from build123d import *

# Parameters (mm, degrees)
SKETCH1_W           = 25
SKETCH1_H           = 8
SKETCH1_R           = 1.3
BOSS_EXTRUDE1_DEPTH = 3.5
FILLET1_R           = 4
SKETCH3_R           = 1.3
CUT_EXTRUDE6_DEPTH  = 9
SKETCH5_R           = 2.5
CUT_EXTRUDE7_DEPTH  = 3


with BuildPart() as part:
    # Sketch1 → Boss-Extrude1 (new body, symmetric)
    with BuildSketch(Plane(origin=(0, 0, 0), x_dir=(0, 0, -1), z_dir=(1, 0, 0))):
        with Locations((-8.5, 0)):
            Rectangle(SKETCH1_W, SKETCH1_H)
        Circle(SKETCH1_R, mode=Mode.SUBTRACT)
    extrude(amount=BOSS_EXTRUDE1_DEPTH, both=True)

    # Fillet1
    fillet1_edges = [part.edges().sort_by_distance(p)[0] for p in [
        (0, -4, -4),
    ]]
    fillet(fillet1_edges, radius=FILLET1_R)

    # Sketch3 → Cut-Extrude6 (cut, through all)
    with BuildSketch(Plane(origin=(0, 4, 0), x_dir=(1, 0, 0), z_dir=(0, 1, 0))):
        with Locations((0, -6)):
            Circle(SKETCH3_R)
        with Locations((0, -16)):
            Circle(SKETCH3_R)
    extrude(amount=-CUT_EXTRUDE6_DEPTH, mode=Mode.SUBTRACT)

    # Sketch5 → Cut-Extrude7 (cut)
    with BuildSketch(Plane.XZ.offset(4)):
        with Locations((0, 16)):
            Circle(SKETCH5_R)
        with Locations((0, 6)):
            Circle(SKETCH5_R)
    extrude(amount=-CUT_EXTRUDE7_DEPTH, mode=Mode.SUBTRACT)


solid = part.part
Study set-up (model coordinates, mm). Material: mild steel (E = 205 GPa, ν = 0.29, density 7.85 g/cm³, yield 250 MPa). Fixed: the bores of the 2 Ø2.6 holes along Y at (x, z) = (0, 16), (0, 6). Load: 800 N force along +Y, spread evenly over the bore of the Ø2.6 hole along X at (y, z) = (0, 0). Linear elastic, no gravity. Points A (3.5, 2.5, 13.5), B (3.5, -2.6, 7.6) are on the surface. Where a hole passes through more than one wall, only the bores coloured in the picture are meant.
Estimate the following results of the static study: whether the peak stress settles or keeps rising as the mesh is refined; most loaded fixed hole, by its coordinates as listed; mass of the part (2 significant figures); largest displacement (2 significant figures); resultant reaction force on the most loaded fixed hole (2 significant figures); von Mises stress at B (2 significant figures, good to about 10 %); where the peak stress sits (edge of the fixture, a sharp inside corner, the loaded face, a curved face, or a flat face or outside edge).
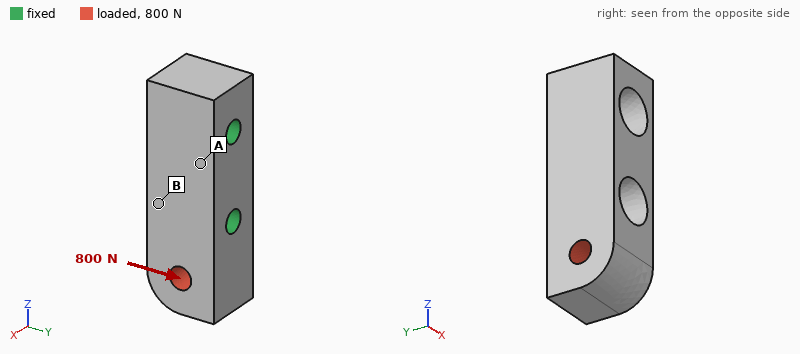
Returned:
keeps rising
(0, 6)
9.2 g
6.2 µm
950 N
45 MPa
edge of the fixture
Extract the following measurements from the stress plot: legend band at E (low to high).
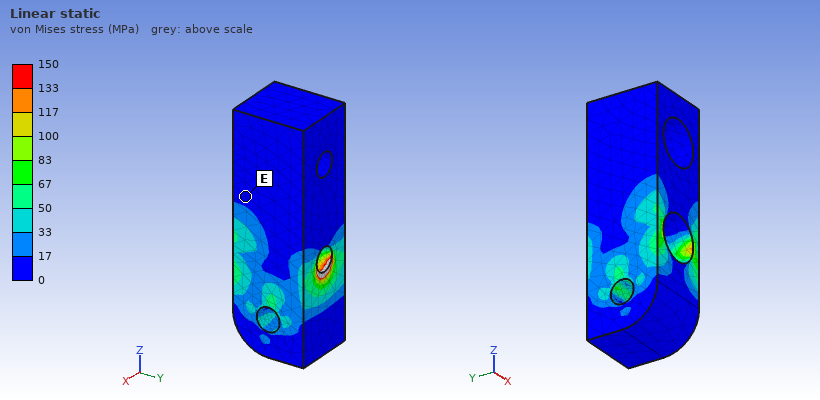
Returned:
0 to 17 MPa
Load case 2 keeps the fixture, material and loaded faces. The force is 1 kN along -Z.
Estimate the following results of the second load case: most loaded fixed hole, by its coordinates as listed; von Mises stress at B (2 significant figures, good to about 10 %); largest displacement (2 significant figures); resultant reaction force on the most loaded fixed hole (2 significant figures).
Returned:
(0, 6)
25 MPa
1.9 µm
860 N
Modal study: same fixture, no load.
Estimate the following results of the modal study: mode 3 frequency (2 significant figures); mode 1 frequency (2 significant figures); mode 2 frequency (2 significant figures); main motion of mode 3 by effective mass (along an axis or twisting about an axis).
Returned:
59 kHz
37 kHz
38 kHz
twisting about Z
